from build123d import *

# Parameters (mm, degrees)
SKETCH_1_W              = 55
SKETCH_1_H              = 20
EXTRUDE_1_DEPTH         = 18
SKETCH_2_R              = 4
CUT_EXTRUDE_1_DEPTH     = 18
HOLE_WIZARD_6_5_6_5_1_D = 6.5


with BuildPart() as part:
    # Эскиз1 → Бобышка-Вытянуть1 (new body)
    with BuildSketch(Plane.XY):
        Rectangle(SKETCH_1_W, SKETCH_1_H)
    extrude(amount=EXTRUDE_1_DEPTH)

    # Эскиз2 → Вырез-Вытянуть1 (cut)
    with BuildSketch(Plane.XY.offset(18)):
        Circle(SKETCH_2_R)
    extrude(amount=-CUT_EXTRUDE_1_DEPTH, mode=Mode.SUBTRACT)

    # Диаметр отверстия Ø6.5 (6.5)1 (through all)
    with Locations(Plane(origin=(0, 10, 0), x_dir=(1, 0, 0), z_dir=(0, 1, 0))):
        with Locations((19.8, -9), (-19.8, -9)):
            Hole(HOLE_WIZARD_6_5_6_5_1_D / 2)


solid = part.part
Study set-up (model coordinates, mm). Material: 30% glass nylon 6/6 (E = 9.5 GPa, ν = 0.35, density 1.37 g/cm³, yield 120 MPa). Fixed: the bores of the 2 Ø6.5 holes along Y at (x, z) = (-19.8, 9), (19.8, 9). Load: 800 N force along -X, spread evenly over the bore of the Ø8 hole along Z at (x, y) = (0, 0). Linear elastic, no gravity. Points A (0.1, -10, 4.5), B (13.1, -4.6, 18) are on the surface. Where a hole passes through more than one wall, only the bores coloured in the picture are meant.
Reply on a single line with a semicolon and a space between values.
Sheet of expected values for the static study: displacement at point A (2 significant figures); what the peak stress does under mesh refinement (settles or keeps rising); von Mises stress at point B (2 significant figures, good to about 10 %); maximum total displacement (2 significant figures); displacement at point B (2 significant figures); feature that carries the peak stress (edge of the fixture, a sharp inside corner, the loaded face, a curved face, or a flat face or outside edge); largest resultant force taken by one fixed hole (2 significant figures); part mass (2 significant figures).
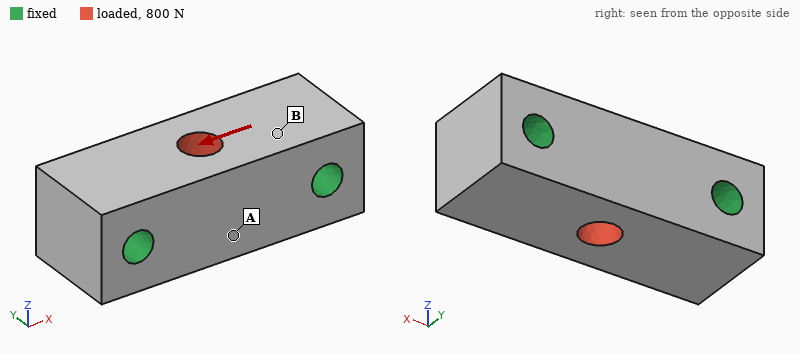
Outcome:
1.4 µm; keeps rising; 0.78 MPa; 2.7 µm; 1.1 µm; edge of the fixture; 400 N; 24 g
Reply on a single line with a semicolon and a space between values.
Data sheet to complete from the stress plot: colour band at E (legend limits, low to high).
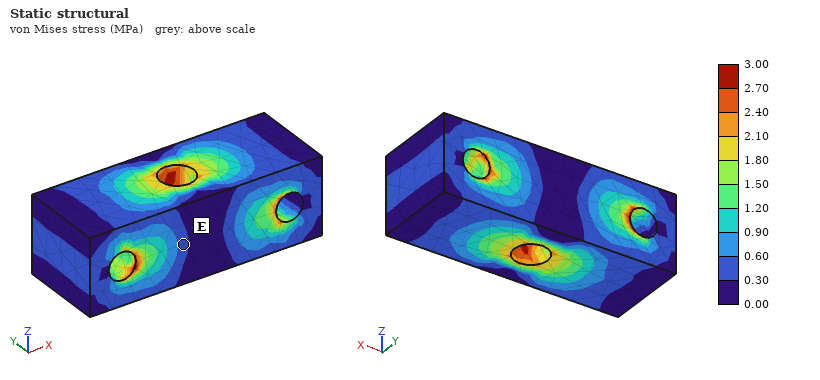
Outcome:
0.30 to 0.60 MPa
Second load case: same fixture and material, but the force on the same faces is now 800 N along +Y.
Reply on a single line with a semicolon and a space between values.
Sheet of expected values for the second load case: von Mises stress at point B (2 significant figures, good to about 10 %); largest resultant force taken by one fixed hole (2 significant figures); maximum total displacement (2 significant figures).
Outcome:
1.9 MPa; 400 N; 8.7 µm
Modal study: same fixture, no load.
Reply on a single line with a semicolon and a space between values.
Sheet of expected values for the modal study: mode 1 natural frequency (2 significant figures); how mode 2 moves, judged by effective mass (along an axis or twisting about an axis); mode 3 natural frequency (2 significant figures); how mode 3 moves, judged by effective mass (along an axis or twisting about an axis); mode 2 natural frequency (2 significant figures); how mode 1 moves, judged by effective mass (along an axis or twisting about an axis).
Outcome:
16 kHz; along Y; 20 kHz; twisting about X; 19 kHz; along Z
